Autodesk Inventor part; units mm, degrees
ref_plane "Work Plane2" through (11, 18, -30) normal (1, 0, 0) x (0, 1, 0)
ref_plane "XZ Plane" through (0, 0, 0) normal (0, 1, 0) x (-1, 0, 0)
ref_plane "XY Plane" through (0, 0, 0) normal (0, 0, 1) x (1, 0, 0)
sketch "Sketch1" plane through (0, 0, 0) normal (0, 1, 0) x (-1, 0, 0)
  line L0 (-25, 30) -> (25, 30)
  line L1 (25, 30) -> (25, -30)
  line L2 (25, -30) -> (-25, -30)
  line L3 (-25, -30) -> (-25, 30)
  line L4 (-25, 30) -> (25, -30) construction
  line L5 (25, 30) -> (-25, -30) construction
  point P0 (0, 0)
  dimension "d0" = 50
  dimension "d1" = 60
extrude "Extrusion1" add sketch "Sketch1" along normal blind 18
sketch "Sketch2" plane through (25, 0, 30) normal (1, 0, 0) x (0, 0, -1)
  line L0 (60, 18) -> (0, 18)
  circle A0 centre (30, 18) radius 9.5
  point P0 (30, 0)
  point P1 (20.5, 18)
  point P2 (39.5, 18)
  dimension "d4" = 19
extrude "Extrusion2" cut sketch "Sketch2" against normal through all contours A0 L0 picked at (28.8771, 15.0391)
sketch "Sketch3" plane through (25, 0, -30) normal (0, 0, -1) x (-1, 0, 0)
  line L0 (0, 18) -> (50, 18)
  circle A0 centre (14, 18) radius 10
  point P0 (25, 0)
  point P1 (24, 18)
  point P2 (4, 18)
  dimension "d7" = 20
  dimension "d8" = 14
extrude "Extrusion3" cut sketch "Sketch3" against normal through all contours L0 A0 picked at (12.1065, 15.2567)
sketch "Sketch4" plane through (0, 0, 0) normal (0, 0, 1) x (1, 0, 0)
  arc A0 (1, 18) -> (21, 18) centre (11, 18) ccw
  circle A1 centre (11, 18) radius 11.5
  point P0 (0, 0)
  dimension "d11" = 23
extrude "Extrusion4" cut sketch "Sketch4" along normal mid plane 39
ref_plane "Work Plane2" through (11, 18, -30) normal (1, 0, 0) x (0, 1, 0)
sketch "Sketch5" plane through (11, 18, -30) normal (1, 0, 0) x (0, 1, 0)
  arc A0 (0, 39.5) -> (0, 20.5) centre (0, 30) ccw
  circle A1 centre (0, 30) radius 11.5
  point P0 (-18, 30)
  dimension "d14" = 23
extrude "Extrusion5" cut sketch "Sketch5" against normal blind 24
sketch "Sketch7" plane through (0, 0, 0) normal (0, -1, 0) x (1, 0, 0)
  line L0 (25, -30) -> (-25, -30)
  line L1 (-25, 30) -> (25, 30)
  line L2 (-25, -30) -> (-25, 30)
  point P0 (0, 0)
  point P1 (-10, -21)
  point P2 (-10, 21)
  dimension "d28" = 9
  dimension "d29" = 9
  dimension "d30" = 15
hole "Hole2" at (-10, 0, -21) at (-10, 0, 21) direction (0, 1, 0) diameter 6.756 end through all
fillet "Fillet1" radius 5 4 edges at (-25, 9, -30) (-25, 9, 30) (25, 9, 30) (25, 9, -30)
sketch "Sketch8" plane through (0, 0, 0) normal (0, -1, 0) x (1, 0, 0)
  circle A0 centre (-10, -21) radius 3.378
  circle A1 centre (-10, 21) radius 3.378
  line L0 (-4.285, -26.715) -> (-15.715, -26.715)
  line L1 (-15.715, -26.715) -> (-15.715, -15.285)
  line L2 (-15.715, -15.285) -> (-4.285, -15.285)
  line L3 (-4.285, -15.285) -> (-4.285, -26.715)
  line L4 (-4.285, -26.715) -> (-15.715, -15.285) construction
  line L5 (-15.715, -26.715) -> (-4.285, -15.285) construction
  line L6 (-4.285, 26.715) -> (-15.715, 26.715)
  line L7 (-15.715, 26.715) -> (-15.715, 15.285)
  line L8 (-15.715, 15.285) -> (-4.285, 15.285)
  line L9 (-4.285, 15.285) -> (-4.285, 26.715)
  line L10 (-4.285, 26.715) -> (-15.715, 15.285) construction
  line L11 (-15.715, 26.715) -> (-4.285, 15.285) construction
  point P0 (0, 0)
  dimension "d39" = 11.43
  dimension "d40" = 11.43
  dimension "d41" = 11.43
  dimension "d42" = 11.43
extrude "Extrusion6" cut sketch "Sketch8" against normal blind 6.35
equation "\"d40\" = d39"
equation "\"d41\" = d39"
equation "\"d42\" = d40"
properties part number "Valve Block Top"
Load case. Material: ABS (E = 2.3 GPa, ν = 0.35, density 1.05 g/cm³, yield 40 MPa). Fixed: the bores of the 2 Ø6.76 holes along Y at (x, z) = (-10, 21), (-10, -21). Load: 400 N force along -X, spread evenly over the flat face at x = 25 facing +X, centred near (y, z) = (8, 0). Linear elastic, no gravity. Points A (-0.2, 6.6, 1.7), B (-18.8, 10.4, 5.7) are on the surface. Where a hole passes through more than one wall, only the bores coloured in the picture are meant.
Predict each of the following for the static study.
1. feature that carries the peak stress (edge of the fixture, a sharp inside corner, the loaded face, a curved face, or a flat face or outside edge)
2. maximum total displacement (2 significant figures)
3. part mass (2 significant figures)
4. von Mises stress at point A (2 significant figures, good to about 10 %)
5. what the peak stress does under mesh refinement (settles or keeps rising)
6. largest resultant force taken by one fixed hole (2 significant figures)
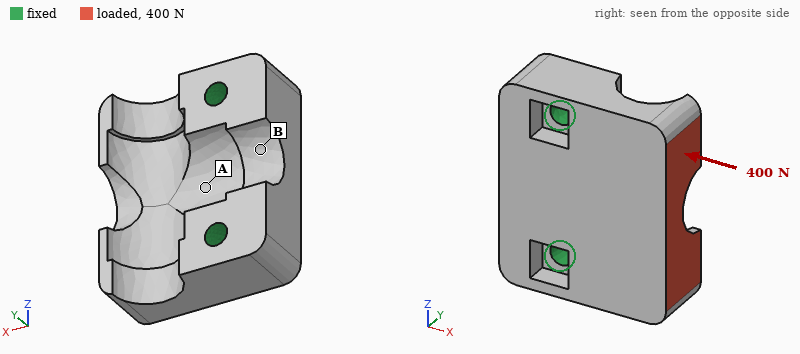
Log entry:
a sharp inside corner
0.15 mm
36 g
1.3 MPa
keeps rising
200 N
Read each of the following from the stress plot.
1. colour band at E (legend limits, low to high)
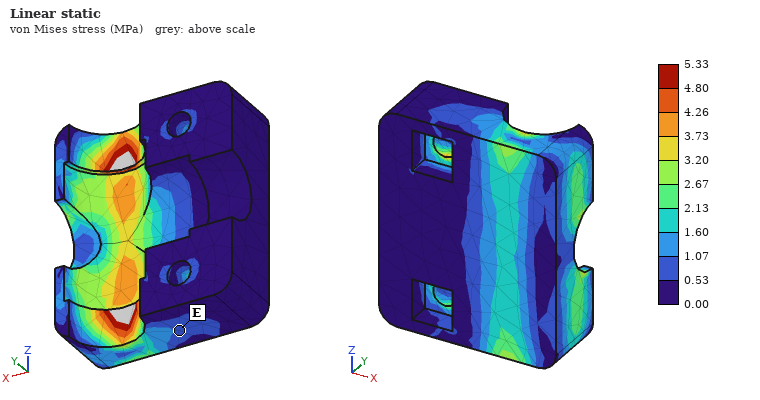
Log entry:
0.53 to 1.07 MPa
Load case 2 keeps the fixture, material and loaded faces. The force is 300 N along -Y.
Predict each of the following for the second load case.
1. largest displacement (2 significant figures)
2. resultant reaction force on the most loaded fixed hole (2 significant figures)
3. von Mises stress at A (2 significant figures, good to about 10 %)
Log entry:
0.55 mm
160 N
3.3 MPa
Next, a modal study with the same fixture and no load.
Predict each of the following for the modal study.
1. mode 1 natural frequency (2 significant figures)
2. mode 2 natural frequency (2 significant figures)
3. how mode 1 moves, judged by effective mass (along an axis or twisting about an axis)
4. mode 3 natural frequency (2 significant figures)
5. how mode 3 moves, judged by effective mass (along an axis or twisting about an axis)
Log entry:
1700 Hz
2500 Hz
along Y
4300 Hz
along Z
